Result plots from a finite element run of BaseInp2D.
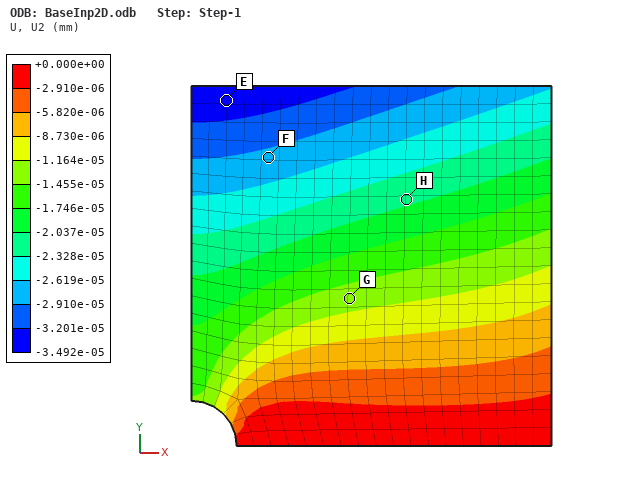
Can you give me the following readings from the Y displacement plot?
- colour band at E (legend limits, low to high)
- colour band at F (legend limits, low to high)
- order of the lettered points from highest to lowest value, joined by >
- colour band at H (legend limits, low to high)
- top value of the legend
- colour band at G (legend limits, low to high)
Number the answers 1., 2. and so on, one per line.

1. -3.492e-05 to -3.201e-05 mm
2. -2.910e-05 to -2.619e-05 mm
3. G > H > F > E
4. -2.328e-05 to -2.037e-05 mm
5. +0.000e+00 mm
6. -1.455e-05 to -1.164e-05 mm
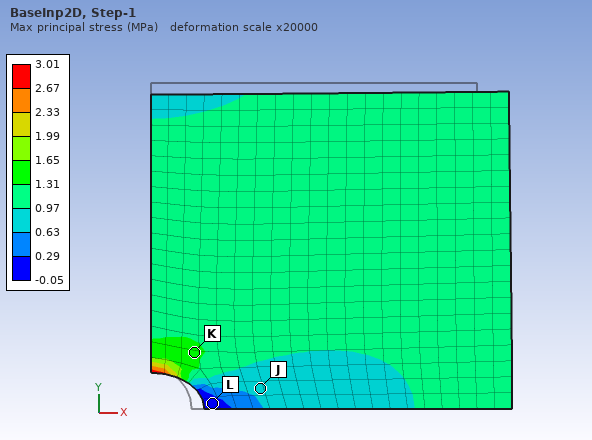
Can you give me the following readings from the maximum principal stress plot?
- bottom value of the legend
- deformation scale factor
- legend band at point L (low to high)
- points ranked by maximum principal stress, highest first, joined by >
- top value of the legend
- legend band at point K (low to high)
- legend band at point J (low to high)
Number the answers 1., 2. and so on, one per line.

1. -0.05 MPa
2. 20000
3. -0.05 to 0.29 MPa
4. K > J > L
5. 3.01 MPa
6. 1.31 to 1.65 MPa
7. 0.63 to 0.97 MPa
